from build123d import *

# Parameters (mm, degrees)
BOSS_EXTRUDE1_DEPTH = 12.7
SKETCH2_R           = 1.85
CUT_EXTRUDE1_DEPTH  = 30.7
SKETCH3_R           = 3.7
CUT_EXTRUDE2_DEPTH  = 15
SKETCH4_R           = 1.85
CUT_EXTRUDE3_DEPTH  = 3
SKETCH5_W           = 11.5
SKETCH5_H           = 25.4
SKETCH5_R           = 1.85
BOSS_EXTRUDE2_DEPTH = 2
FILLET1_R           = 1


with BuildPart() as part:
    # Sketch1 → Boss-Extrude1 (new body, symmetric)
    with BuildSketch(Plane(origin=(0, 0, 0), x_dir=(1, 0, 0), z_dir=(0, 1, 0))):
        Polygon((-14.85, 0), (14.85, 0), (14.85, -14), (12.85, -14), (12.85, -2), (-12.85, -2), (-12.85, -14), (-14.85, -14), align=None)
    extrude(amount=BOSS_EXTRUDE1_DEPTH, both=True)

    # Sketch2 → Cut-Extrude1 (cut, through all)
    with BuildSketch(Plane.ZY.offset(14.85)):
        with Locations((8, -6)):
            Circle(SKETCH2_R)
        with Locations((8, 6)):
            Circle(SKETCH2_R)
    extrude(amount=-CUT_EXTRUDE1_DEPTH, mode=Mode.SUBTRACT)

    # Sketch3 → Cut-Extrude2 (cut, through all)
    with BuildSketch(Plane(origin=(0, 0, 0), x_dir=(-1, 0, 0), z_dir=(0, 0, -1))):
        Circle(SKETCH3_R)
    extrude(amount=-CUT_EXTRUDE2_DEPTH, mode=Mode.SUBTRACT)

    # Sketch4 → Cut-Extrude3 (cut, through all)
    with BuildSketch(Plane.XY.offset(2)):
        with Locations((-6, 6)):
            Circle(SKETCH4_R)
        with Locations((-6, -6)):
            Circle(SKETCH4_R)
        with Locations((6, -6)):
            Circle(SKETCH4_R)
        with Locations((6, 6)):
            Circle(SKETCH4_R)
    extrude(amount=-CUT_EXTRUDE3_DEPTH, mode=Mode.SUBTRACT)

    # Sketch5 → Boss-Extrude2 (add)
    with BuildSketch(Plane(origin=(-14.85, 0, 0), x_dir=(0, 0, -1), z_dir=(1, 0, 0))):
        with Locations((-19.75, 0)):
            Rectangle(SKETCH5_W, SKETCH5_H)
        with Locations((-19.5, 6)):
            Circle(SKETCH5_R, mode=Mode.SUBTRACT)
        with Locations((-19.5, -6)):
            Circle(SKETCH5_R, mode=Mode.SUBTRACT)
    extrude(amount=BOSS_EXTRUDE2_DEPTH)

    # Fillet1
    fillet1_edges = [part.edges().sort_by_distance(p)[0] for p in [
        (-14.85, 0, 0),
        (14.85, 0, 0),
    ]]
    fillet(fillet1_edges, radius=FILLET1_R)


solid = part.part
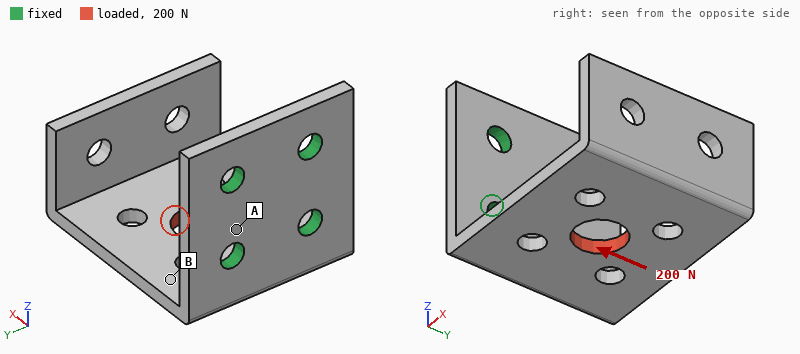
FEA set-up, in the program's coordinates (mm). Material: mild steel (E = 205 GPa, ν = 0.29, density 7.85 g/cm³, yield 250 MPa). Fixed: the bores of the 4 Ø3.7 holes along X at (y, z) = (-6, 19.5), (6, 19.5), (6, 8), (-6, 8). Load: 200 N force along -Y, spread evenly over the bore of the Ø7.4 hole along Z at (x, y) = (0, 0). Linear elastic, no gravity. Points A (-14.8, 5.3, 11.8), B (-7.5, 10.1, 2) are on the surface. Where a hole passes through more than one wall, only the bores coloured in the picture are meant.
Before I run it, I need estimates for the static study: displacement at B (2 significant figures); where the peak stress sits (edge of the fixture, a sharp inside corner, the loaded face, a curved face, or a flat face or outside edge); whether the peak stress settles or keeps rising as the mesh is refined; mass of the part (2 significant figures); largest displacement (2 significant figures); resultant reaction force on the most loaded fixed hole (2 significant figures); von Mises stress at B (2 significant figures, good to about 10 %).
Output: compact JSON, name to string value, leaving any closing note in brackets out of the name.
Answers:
{"displacement at B": "11 µm", "where the peak stress sits": "edge of the fixture", "whether the peak stress settles or keeps rising as the mesh is refined": "keeps rising", "mass of the part": "24 g", "largest displacement": "37 µm", "resultant reaction force on the most loaded fixed hole": "230 N", "von Mises stress at B": "29 MPa"}
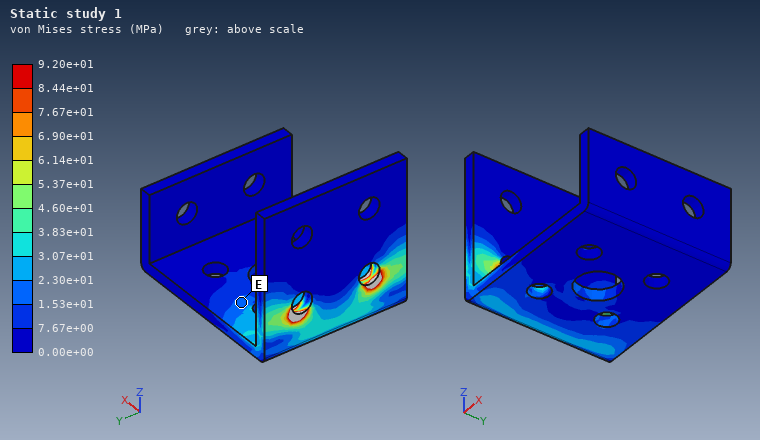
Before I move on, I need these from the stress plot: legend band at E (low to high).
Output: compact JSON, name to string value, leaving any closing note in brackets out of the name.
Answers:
{"legend band at E": "1.53e+01 to 2.30e+01 MPa"}
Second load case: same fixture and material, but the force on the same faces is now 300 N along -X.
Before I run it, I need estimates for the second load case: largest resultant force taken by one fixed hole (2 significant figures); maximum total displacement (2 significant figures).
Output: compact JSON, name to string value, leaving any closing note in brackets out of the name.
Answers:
{"largest resultant force taken by one fixed hole": "160 N", "maximum total displacement": "47 µm"}
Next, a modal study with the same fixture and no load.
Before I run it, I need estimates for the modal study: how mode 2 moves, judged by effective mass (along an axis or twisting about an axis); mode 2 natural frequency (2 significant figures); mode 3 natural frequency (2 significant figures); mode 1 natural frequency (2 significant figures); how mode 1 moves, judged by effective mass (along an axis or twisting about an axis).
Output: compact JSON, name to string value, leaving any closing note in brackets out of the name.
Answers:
{"how mode 2 moves, judged by effective mass": "along Y", "mode 2 natural frequency": "2200 Hz", "mode 3 natural frequency": "4200 Hz", "mode 1 natural frequency": "940 Hz", "how mode 1 moves, judged by effective mass": "along Z"}
